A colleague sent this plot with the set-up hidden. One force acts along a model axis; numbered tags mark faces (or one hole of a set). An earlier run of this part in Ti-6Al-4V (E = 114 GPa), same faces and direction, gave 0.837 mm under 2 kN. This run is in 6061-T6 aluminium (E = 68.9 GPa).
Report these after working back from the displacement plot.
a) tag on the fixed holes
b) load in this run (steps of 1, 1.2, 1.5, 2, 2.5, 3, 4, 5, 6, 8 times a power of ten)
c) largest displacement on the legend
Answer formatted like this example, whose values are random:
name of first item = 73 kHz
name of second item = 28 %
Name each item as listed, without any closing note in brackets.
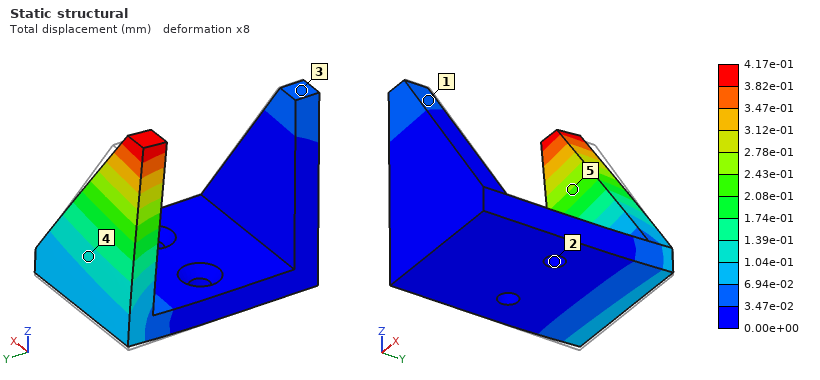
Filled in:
tag on the fixed holes = 2
load in this run = 600 N
largest displacement on the legend = 4.17e-01 mm
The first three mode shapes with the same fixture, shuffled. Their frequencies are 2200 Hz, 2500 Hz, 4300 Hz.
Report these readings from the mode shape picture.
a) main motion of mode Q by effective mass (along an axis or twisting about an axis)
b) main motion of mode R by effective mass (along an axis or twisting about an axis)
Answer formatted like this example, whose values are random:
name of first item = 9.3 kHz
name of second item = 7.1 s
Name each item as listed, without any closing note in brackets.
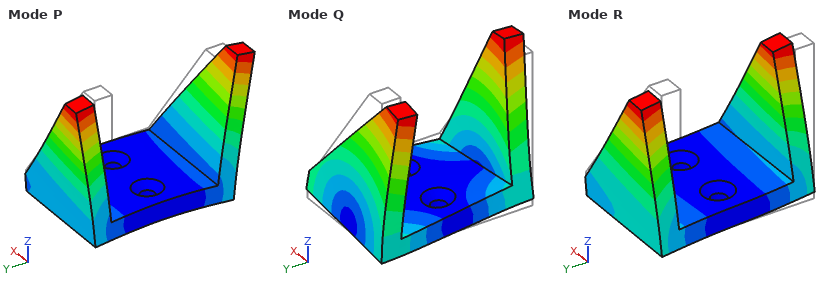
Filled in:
main motion of mode Q by effective mass = twisting about Z
main motion of mode R by effective mass = along Y
